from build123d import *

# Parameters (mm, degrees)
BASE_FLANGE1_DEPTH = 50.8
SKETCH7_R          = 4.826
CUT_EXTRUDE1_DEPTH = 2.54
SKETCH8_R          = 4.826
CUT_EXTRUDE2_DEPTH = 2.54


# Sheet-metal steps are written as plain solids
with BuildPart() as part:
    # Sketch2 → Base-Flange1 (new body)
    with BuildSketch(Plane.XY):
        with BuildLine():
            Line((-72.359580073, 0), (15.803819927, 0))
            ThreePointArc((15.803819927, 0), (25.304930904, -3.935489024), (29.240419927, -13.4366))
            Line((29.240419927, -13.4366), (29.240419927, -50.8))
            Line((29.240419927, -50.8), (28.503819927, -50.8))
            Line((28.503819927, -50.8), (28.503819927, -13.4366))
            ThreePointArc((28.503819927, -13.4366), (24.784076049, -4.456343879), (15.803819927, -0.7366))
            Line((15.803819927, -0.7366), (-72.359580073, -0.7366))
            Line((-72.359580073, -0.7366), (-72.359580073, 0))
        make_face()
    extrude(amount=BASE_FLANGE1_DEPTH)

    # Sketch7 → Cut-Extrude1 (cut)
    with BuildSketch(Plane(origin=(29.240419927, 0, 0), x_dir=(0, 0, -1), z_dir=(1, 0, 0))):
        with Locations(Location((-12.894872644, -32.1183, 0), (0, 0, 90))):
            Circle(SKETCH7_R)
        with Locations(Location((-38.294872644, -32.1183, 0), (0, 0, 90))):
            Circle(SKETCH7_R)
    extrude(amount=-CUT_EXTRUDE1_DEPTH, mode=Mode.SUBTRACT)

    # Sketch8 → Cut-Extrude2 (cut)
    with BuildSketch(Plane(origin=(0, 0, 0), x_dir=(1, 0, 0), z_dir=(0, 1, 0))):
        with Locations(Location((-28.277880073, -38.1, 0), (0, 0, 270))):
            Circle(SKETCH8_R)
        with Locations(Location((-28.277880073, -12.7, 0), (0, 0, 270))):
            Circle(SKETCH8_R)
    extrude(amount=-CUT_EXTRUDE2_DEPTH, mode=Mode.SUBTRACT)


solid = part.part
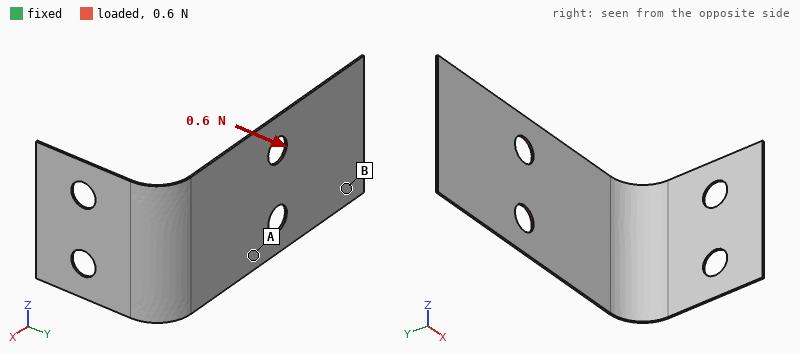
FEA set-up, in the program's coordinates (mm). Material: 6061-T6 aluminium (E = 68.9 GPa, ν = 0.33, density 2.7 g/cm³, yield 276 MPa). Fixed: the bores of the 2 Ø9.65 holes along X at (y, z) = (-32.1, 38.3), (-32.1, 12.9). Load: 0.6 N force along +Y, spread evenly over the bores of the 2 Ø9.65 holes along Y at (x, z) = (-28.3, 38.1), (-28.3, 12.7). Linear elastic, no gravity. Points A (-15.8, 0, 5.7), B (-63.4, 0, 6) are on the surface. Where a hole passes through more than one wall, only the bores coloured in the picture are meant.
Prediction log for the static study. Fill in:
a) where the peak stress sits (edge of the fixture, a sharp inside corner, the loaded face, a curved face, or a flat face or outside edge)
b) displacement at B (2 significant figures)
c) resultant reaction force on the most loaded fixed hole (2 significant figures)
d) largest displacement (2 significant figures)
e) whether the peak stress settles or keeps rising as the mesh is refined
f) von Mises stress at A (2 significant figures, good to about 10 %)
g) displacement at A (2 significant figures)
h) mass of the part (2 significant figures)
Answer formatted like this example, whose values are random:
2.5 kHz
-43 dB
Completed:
edge of the fixture
1.1 mm
0.37 N
1.2 mm
keeps rising
1.7 MPa
0.47 mm
14 g
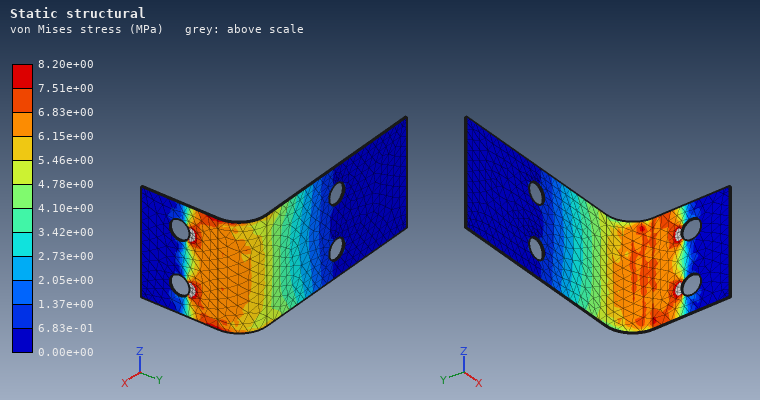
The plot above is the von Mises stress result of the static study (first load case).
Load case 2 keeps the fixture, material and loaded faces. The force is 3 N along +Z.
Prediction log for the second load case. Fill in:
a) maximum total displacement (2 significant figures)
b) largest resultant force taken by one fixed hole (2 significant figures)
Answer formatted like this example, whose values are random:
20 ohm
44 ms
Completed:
1.2 mm
6.2 N
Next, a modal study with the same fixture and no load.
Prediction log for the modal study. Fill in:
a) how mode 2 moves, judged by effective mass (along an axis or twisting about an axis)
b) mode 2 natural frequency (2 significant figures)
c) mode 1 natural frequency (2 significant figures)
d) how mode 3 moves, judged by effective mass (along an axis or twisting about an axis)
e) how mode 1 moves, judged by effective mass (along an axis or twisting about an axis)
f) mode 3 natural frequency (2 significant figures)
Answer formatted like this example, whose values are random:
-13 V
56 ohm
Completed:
along Z
100 Hz
44 Hz
along X
along Y
230 Hz
